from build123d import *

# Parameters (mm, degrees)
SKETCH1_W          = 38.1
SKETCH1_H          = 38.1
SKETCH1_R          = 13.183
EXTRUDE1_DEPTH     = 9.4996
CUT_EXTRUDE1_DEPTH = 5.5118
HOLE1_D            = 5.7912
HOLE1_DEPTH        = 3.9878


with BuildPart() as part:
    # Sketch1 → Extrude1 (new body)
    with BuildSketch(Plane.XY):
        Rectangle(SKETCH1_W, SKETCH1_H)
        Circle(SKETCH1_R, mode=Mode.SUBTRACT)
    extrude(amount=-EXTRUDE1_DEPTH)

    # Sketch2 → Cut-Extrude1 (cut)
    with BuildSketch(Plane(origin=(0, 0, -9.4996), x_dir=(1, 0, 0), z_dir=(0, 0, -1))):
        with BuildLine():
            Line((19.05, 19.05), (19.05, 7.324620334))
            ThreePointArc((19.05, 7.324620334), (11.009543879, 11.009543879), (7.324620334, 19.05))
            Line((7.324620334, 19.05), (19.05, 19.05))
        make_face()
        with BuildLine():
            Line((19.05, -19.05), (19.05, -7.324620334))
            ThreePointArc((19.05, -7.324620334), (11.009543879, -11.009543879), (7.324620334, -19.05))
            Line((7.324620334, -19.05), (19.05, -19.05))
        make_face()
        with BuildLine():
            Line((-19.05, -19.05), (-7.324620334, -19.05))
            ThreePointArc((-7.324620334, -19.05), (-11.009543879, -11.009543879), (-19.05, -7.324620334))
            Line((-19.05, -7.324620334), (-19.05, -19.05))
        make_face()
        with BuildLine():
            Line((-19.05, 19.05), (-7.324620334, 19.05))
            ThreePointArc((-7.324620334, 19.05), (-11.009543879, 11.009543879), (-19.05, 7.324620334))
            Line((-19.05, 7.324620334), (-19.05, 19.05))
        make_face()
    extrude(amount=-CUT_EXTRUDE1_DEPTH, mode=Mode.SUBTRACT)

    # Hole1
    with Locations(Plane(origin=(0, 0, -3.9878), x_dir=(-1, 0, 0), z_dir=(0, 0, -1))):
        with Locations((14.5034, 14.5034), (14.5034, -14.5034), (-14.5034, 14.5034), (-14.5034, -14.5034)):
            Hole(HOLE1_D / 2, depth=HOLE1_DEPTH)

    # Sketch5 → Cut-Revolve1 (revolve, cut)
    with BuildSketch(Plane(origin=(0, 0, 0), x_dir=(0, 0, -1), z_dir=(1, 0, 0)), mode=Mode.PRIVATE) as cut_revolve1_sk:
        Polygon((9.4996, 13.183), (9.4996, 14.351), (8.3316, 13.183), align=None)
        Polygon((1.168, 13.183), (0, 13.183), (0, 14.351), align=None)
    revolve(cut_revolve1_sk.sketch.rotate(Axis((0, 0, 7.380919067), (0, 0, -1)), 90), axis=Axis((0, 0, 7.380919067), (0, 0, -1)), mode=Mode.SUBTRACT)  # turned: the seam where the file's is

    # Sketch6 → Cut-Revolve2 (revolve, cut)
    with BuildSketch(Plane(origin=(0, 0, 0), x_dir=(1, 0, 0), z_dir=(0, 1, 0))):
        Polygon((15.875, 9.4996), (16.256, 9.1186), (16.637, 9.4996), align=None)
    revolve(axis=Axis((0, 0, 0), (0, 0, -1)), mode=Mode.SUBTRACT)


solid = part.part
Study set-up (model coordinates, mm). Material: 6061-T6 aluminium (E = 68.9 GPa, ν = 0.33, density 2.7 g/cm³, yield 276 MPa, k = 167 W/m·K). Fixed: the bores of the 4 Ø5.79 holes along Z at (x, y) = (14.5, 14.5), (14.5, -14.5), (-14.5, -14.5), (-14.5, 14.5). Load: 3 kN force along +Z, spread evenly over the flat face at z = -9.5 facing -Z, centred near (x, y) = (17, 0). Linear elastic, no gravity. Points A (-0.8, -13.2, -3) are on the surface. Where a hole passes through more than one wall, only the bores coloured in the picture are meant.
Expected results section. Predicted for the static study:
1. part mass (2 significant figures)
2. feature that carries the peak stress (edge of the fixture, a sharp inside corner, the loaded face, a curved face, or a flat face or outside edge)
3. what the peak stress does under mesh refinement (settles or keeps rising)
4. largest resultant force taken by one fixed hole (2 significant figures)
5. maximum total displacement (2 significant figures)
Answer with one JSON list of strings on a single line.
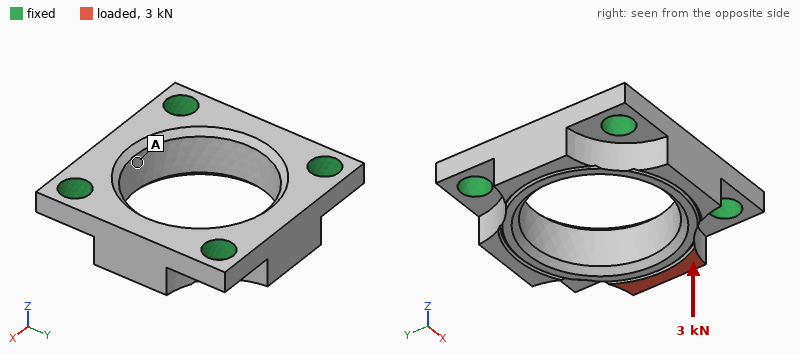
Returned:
["16 g", "edge of the fixture", "keeps rising", "1.7 kN", "50 µm"]
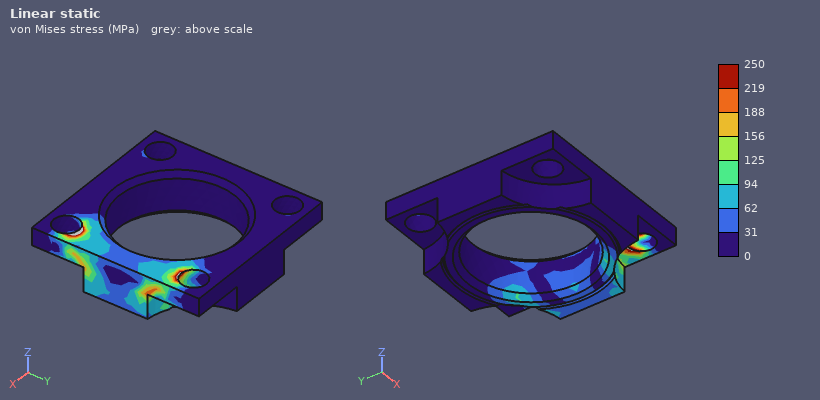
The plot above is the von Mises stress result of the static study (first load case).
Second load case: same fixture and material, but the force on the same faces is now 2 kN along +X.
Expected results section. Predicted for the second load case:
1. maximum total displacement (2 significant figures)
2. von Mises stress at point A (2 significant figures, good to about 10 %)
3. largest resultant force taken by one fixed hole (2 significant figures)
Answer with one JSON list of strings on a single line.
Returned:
["48 µm", "19 MPa", "930 N"]
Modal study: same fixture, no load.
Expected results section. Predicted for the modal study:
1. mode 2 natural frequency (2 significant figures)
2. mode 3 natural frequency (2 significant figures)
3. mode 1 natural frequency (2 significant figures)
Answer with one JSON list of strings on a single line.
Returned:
["32 kHz", "32 kHz", "25 kHz"]
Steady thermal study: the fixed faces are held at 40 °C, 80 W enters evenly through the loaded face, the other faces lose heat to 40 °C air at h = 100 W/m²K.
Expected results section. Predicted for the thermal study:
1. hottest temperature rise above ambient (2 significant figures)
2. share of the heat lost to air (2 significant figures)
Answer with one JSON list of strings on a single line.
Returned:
["75 K", "4.0 %"]
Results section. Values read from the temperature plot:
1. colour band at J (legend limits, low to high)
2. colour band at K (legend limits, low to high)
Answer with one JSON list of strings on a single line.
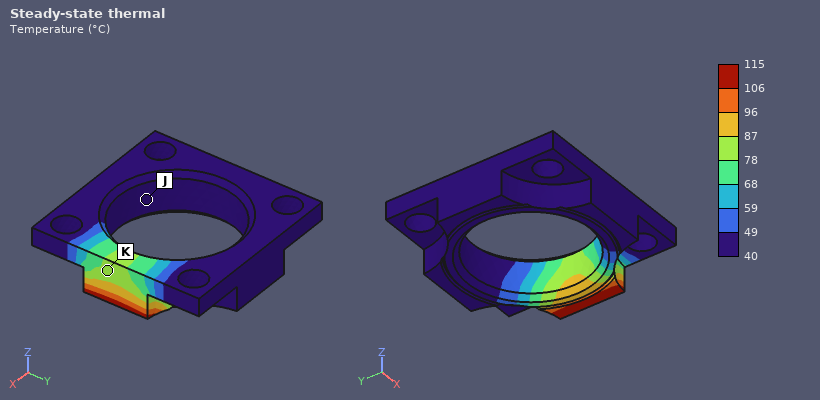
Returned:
["40 to 49 °C", "78 to 87 °C"]
